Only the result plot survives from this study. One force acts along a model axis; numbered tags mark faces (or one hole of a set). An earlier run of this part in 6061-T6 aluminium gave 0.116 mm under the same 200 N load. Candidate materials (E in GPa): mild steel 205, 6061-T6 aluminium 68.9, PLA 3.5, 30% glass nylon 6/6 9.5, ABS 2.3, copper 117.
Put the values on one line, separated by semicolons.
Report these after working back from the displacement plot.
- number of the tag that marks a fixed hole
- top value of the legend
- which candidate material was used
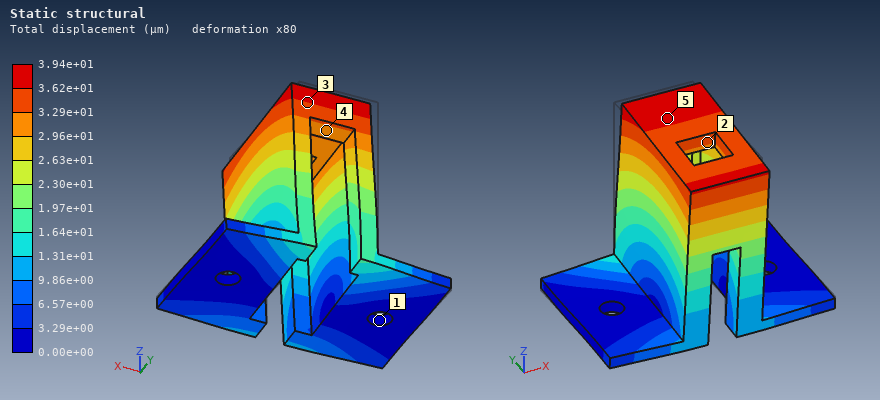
1; 3.94e+01 µm; mild steel
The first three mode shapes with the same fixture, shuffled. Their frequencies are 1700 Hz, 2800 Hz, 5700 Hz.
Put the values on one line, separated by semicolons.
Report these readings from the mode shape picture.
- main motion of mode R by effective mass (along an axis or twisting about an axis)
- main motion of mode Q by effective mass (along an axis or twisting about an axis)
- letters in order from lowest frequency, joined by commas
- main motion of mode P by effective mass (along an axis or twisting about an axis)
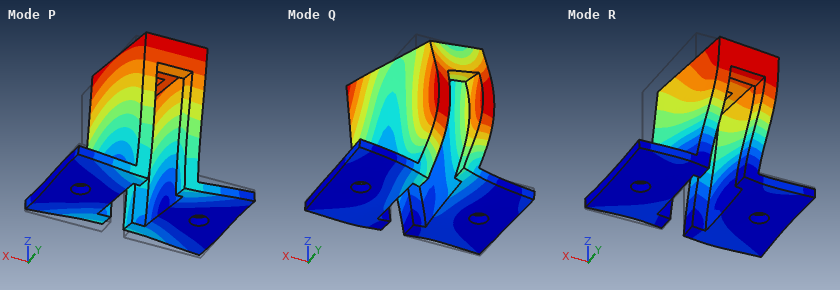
along X; twisting about Z; P, R, Q; along Y
